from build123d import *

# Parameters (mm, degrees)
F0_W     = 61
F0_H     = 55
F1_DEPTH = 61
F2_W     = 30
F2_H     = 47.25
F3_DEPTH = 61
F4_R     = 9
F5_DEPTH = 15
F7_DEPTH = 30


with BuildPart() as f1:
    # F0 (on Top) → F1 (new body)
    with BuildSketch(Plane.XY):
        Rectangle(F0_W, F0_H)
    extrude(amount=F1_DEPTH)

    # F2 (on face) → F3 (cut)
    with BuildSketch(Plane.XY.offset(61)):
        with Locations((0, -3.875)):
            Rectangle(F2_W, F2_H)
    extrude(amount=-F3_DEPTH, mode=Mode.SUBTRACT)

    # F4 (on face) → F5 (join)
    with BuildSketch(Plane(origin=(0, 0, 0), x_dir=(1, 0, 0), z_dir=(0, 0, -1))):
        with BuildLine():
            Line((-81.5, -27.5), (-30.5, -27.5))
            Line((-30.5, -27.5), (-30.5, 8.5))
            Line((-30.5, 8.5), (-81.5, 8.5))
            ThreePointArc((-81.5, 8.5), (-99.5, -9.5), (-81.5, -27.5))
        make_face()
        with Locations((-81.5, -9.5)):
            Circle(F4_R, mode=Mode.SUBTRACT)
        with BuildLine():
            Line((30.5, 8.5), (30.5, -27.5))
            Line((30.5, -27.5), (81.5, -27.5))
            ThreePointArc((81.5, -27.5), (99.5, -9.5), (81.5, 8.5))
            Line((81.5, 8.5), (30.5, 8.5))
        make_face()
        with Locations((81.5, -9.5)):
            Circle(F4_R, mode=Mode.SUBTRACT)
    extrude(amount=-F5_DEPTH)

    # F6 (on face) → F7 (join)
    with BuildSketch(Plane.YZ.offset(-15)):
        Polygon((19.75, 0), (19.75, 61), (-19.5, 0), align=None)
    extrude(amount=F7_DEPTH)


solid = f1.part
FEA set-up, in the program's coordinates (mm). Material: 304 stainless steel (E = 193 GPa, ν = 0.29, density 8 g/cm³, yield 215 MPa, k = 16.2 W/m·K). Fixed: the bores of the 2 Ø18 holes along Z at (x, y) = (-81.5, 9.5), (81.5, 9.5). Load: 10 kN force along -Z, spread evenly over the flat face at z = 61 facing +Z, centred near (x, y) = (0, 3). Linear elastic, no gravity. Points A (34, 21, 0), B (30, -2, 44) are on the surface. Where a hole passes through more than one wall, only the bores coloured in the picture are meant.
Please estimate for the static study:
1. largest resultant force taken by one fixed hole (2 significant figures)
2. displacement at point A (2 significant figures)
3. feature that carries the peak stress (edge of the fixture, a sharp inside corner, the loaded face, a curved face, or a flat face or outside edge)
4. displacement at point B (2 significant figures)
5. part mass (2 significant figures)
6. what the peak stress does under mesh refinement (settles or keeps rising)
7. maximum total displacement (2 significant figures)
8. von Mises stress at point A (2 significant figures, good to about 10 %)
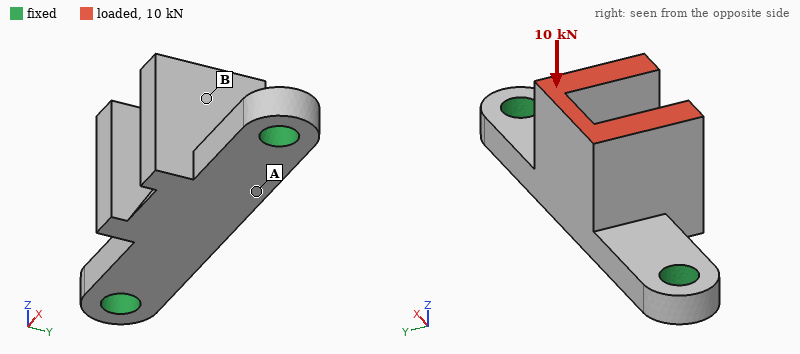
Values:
5.5 kN
27 µm
edge of the fixture
52 µm
1.7 kg
keeps rising
72 µm
41 MPa
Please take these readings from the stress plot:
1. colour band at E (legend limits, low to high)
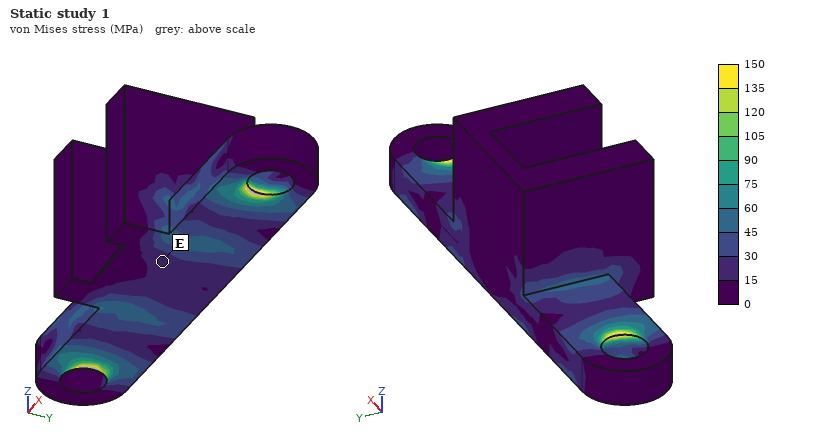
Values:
15 to 30 MPa
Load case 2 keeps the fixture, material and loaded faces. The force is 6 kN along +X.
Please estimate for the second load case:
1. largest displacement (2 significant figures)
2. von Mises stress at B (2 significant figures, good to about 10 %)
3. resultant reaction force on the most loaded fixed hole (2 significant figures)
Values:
41 µm
16 MPa
4.2 kN
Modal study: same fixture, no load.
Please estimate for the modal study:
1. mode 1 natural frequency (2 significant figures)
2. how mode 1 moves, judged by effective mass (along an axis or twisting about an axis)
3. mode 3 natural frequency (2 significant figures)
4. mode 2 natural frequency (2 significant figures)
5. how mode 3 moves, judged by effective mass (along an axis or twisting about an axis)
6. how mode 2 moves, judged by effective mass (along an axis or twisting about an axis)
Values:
1400 Hz
along Y
3400 Hz
2200 Hz
along X
along Z
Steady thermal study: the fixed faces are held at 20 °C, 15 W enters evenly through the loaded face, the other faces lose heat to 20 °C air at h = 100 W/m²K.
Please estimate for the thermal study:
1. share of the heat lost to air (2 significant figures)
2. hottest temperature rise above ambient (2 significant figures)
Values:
95 %
15 K
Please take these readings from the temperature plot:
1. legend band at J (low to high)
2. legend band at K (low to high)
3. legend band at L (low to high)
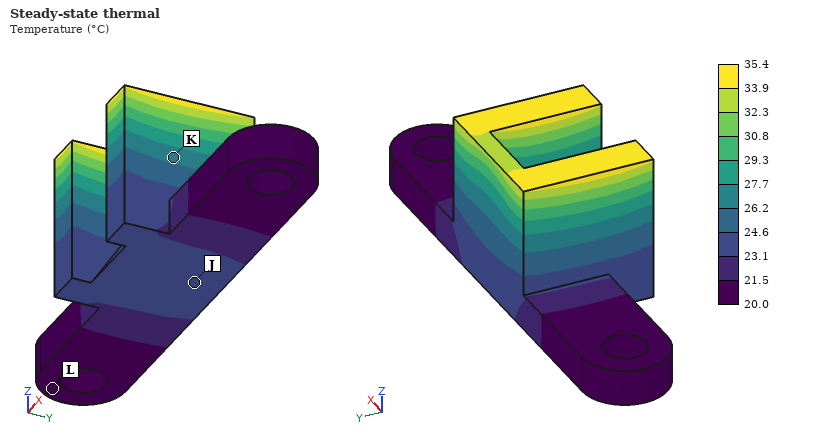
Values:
23.1 to 24.6 °C
26.2 to 27.7 °C
20.0 to 21.5 °C
